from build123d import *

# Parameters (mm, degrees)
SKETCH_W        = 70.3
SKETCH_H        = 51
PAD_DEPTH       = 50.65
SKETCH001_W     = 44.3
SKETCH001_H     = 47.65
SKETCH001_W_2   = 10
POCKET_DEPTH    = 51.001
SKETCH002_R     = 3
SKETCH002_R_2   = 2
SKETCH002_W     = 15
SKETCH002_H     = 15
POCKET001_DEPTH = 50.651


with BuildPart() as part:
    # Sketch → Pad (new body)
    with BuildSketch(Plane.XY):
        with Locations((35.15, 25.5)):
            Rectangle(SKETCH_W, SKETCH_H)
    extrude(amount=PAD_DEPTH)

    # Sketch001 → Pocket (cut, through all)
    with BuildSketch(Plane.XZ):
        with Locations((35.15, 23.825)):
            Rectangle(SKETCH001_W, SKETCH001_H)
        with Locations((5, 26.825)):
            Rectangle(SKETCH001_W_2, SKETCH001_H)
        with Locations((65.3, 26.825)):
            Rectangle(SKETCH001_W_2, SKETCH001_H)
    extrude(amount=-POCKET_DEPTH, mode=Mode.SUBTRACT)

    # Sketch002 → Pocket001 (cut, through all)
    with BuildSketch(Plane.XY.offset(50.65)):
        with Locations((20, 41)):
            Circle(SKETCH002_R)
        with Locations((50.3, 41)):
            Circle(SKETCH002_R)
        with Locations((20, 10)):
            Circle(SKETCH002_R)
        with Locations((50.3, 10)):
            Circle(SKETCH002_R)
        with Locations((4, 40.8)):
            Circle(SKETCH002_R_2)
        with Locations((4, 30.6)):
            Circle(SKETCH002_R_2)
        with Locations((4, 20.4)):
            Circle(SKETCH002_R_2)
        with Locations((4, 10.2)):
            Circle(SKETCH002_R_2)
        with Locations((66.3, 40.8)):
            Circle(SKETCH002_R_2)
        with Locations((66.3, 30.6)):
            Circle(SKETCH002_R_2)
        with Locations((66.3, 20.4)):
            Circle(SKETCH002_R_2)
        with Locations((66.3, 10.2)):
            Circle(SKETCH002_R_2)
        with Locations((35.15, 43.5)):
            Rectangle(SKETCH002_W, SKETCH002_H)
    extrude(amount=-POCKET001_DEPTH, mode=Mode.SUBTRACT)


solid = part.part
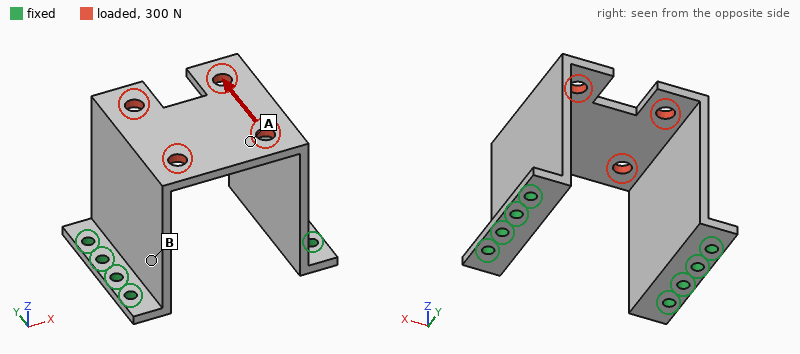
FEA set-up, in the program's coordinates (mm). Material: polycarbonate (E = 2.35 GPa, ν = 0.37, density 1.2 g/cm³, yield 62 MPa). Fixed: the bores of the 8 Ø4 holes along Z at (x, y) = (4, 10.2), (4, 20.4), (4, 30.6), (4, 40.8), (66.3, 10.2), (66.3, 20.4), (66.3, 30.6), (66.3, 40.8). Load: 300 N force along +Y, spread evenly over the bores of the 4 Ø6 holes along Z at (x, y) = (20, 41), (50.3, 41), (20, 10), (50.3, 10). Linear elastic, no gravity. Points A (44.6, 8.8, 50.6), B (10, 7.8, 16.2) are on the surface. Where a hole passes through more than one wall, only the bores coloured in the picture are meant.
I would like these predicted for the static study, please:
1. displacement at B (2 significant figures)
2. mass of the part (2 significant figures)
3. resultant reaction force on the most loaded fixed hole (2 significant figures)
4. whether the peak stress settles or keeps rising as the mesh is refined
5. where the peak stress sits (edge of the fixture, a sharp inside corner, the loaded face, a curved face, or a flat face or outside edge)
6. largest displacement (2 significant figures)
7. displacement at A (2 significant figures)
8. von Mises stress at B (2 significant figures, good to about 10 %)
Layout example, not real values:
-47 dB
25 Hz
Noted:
0.37 mm
29 g
200 N
keeps rising
edge of the fixture
0.82 mm
0.78 mm
6.7 MPa
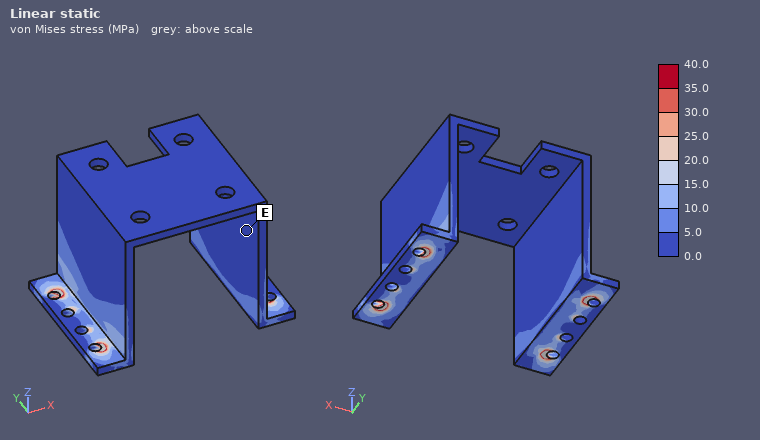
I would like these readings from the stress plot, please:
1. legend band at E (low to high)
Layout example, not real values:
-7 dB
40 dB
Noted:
0.0 to 5.0 MPa
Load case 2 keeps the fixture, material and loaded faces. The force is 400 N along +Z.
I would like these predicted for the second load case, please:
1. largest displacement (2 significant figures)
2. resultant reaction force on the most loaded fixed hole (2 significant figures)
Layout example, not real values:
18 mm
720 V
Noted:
1.1 mm
58 N
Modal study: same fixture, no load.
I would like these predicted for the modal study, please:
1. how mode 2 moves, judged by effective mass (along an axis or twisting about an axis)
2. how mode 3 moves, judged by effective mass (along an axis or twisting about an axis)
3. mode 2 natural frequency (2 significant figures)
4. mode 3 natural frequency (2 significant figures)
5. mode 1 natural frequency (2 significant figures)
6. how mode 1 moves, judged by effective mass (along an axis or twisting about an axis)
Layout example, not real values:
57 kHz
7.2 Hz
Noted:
twisting about Z
along Y
770 Hz
820 Hz
260 Hz
along X
